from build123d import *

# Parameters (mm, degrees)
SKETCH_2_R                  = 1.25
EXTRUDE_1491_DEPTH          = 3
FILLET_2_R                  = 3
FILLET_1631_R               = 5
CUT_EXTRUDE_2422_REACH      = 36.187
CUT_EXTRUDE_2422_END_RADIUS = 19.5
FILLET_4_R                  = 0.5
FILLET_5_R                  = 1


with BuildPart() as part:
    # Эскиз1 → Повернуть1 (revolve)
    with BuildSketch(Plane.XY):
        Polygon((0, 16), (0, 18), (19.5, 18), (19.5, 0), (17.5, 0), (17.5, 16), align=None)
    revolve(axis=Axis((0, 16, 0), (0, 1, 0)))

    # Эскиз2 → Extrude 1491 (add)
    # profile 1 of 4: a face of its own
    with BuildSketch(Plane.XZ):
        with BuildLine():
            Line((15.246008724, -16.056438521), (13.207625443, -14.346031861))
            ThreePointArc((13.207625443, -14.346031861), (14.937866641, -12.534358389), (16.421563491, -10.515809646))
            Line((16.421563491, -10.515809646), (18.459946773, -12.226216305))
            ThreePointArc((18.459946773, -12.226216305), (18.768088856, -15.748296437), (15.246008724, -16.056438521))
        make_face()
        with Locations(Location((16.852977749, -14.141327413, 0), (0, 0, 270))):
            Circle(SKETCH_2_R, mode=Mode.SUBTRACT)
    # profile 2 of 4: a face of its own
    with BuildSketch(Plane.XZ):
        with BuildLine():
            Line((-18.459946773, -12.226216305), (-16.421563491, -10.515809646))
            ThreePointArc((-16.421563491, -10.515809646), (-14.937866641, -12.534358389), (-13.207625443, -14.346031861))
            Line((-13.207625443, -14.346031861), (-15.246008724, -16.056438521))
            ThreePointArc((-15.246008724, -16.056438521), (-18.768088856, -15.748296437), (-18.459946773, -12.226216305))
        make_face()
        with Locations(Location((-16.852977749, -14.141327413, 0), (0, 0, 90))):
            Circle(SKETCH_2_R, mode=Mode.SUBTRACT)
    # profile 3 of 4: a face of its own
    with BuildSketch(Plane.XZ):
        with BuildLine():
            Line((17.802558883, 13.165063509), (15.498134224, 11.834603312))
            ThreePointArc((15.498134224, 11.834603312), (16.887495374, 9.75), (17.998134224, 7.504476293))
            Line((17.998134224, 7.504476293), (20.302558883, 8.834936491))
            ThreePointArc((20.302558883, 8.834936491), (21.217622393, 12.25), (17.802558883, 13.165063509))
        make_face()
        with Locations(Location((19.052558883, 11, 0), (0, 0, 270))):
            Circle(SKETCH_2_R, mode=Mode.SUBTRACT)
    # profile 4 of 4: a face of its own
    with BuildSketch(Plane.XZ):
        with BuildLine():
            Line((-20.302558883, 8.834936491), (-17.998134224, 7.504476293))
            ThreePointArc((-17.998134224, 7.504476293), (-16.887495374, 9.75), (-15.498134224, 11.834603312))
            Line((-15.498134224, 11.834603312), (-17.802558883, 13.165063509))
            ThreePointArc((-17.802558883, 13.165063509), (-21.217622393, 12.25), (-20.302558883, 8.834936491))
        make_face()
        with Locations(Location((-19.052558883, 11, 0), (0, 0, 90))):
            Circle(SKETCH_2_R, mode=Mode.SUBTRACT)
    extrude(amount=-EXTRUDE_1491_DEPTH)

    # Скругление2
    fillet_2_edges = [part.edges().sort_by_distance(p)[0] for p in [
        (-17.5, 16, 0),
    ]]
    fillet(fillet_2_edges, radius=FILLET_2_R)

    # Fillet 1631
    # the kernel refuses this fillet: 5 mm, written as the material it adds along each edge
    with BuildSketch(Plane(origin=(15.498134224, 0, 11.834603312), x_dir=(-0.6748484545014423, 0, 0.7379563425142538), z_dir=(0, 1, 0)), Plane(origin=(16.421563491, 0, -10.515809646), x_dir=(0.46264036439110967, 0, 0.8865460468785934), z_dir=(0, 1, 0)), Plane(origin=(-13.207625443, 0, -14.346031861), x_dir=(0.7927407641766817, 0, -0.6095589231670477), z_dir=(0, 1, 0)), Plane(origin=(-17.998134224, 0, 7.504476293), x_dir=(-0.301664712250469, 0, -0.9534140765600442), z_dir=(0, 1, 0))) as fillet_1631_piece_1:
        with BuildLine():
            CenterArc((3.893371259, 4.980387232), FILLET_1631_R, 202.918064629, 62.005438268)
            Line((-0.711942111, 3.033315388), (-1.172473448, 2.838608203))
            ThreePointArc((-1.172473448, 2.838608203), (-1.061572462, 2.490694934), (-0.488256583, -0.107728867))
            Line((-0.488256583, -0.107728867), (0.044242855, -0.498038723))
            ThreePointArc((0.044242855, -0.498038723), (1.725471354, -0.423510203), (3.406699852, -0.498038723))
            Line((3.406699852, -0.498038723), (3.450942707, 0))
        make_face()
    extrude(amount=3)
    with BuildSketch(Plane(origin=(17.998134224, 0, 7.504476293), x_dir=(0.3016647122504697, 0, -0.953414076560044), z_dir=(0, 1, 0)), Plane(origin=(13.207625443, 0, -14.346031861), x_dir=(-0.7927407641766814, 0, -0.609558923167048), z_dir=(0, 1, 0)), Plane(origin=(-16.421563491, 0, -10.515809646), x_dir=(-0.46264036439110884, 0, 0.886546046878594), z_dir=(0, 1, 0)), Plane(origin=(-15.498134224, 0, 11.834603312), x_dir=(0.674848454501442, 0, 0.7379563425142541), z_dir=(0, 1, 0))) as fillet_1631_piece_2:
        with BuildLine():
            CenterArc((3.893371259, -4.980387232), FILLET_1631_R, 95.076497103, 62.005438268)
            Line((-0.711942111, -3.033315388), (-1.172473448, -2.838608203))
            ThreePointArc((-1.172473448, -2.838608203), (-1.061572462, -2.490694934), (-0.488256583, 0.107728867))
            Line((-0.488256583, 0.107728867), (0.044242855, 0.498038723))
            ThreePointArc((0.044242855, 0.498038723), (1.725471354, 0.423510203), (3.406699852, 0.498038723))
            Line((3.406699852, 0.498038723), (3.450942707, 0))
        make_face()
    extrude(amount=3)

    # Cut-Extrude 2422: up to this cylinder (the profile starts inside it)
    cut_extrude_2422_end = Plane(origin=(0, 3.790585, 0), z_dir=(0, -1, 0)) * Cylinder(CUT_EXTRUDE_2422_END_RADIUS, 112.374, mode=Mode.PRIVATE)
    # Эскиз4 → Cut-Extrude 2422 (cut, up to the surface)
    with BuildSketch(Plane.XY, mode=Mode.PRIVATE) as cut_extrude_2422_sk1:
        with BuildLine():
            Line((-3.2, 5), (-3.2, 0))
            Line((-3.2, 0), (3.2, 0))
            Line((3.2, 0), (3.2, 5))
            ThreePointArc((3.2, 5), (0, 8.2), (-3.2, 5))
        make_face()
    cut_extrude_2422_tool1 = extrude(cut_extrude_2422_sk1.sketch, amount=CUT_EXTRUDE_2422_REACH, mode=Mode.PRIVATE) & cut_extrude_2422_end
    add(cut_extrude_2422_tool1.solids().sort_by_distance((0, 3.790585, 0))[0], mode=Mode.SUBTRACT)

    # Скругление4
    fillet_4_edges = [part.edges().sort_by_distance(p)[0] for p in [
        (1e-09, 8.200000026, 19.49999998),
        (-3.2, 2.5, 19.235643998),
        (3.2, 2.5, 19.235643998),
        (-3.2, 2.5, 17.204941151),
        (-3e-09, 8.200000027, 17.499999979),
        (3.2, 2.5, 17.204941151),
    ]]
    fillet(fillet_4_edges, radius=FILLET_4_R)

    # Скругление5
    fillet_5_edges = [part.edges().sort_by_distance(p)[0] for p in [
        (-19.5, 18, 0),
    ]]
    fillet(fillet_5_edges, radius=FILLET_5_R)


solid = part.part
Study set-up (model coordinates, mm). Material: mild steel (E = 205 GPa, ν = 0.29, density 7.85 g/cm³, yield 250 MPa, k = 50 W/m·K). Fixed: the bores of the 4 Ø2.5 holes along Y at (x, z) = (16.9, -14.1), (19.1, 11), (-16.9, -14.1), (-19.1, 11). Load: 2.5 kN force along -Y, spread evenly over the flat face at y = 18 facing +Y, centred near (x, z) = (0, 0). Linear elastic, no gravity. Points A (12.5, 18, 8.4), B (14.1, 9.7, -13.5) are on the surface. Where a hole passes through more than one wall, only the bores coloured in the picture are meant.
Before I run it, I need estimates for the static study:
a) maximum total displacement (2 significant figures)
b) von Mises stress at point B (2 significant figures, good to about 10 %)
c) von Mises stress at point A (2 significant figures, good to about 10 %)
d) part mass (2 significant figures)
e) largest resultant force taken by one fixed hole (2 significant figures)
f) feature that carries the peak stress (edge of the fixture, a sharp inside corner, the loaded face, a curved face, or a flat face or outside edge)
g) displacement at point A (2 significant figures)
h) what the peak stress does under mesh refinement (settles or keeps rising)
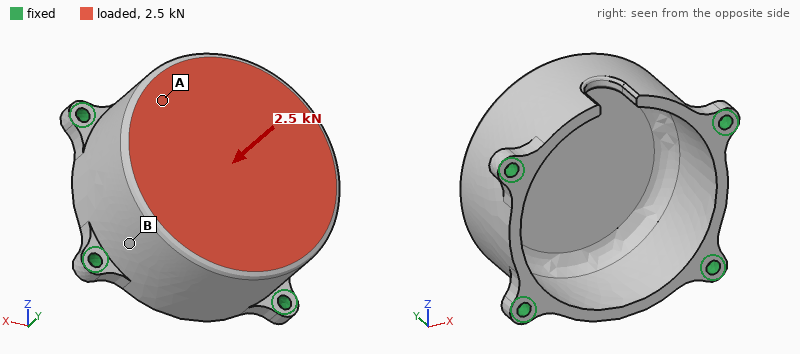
32 µm
21 MPa
58 MPa
51 g
730 N
edge of the fixture
7.8 µm
keeps rising
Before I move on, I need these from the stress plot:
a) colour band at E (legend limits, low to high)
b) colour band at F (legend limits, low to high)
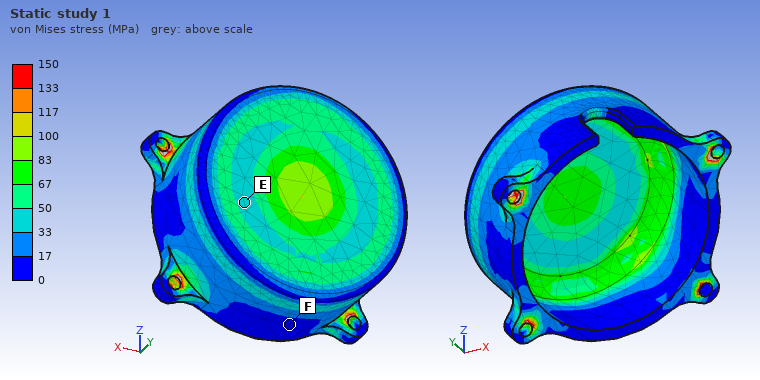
33 to 50 MPa
0 to 17 MPa
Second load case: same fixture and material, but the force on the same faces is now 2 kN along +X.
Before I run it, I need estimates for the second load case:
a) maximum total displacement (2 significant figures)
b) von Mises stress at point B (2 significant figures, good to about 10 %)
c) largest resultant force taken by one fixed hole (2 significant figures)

11 µm
18 MPa
730 N
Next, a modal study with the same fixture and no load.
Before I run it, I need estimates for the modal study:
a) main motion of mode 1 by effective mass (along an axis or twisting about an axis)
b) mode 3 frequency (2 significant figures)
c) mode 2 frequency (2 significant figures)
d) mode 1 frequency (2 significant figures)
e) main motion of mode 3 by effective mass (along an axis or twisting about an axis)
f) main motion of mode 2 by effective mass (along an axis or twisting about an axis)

along Z
13 kHz
13 kHz
11 kHz
along Y
along X
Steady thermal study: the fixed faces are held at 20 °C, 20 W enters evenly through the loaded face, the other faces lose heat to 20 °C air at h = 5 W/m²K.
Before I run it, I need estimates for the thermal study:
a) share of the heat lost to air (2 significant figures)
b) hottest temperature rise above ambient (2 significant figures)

4.6 %
60 K
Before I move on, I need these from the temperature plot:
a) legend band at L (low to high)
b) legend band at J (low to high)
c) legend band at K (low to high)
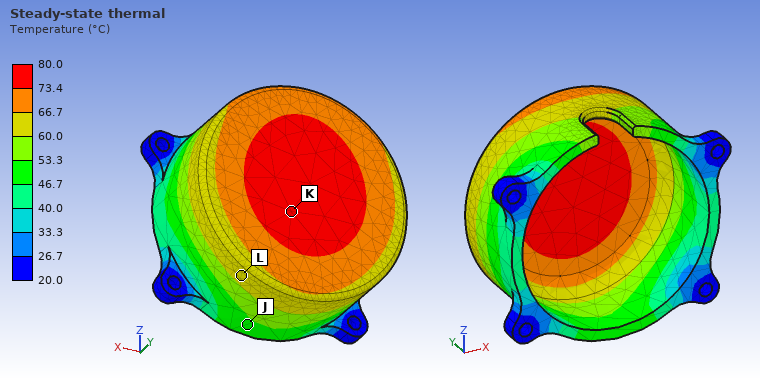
60.0 to 66.7 °C
46.7 to 53.3 °C
73.4 to 80.0 °C
